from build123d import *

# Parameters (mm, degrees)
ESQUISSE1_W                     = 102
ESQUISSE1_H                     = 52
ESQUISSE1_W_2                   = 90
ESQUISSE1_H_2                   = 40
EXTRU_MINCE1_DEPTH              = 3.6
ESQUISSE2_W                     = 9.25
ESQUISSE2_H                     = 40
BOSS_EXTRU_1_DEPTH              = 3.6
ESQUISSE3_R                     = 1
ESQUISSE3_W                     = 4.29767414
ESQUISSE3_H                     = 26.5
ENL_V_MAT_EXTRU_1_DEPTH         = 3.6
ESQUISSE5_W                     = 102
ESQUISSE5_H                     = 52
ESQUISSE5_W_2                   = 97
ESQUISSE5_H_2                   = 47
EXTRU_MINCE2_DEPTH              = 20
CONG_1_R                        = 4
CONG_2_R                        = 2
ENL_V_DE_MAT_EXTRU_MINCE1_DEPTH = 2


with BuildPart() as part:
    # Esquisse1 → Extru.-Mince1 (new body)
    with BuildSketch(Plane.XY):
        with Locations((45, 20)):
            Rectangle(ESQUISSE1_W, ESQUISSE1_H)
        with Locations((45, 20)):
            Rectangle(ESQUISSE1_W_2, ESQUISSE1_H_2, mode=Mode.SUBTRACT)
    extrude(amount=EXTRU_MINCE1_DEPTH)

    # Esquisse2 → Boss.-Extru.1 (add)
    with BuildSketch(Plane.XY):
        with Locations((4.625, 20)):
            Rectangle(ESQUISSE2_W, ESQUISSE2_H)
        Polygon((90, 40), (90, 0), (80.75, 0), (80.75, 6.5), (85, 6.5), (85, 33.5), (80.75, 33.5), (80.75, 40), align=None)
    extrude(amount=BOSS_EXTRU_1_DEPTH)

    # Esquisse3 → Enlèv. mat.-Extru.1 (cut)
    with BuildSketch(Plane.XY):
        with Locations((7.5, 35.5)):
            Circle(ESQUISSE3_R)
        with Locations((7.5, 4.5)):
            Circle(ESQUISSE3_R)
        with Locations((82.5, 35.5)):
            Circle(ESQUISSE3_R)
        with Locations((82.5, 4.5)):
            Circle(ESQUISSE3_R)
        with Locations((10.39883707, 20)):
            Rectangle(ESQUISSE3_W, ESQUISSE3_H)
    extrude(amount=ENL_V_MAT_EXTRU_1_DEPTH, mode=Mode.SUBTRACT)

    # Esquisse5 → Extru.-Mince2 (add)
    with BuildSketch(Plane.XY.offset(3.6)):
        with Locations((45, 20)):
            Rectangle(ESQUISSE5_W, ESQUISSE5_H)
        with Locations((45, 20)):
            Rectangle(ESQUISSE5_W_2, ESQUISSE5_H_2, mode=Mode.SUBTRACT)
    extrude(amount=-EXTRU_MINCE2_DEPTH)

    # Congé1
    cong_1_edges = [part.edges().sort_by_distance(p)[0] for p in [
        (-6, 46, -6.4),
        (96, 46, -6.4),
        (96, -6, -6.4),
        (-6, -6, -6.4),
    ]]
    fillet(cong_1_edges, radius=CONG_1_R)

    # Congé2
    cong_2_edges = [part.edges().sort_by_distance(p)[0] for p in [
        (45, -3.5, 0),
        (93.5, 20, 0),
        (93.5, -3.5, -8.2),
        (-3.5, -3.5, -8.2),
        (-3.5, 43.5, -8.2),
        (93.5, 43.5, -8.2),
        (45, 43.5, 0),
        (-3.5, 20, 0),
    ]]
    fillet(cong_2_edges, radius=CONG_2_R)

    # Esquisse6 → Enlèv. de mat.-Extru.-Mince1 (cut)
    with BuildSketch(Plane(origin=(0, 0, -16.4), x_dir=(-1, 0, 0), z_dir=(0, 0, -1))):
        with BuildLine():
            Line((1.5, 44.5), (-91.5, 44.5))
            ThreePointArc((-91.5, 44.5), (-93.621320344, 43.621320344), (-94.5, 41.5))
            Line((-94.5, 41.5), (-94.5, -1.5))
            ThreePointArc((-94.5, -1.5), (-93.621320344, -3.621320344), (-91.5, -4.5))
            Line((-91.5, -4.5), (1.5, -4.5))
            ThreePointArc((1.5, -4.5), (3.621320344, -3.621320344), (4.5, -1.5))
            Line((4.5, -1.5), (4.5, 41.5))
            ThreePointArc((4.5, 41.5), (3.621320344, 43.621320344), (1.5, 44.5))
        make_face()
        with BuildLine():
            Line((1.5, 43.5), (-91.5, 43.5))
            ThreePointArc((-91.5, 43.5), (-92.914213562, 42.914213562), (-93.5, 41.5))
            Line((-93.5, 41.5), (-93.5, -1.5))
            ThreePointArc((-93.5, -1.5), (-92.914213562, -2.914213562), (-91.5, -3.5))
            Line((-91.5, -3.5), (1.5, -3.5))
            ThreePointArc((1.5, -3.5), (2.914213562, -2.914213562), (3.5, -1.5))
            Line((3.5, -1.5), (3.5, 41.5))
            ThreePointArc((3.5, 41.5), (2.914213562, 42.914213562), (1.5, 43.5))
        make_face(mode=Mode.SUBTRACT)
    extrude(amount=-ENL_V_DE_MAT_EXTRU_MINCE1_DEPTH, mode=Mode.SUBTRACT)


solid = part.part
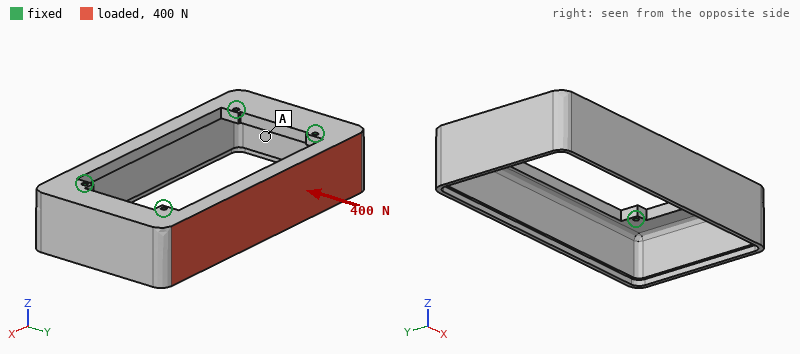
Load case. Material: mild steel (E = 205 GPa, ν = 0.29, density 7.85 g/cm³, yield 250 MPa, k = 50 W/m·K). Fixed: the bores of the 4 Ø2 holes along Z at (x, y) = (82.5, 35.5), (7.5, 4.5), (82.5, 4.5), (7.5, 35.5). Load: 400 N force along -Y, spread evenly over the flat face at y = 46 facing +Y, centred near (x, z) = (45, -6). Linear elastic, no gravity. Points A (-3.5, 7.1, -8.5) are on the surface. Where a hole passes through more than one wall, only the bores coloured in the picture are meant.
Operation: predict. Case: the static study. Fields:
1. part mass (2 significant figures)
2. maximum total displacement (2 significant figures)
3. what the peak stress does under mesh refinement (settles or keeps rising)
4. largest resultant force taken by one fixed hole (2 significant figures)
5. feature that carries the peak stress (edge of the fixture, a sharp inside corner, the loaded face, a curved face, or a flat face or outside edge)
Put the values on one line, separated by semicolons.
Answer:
160 g; 66 µm; keeps rising; 270 N; a sharp inside corner
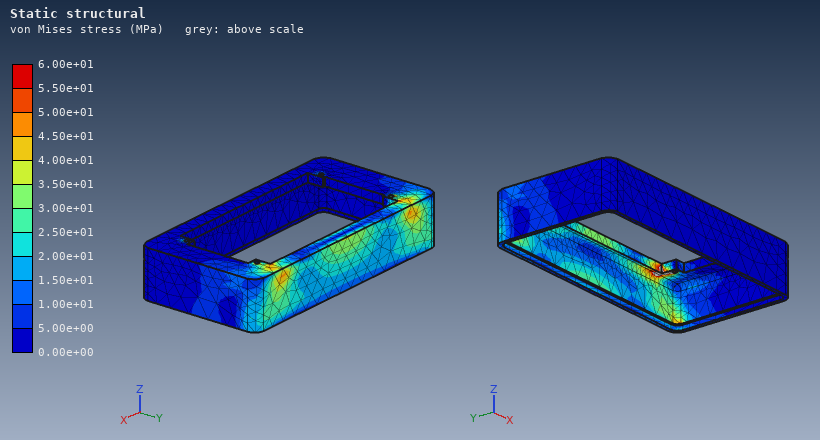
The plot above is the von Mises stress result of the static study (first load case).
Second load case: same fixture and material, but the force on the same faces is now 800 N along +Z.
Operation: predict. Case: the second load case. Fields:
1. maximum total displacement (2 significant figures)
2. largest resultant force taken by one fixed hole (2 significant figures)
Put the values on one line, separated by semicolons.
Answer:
48 µm; 490 N
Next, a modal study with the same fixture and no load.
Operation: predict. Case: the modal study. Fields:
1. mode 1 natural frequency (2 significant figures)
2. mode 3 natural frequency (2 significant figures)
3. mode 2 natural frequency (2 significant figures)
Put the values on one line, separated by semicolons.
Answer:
2700 Hz; 5600 Hz; 2800 Hz
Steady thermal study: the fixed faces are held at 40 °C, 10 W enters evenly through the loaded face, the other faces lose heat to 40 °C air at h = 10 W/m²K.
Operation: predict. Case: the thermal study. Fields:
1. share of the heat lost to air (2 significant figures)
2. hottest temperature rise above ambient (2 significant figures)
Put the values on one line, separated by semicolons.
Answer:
14 %; 43 K
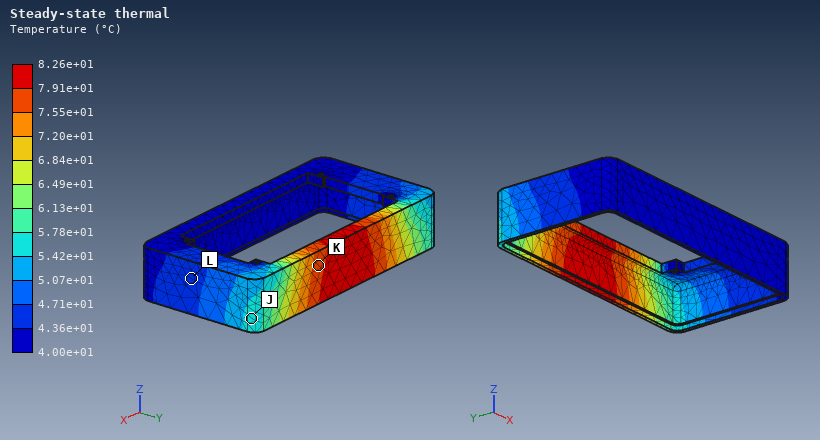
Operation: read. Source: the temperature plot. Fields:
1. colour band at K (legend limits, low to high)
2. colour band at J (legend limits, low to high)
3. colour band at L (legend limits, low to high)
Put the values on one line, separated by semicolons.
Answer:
7.55e+01 to 7.91e+01 °C; 5.42e+01 to 5.78e+01 °C; 4.36e+01 to 4.71e+01 °C
